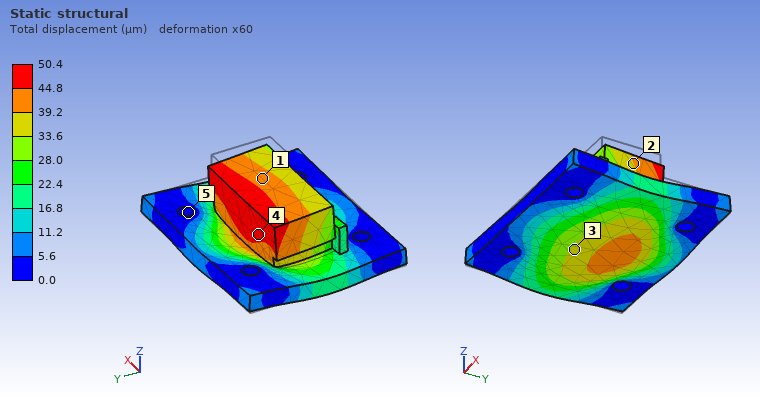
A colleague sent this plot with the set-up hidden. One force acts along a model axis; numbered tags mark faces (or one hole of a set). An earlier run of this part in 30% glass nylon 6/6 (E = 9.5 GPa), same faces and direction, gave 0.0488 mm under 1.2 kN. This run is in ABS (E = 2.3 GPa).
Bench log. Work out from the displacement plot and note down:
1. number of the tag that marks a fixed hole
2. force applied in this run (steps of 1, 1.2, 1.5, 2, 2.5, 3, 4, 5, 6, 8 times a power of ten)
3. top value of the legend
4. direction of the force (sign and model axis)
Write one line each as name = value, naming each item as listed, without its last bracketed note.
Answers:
number of the tag that marks a fixed hole = 5
force applied in this run = 300 N
top value of the legend = 50.4 µm
direction of the force = -Z
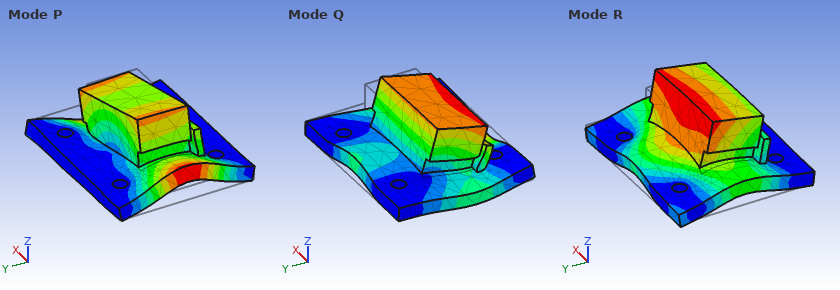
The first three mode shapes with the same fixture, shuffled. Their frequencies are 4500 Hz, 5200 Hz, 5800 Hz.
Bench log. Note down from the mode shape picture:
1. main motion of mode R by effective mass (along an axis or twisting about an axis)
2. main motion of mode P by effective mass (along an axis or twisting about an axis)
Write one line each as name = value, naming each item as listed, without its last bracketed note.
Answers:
main motion of mode R by effective mass = along Z
main motion of mode P by effective mass = along X
